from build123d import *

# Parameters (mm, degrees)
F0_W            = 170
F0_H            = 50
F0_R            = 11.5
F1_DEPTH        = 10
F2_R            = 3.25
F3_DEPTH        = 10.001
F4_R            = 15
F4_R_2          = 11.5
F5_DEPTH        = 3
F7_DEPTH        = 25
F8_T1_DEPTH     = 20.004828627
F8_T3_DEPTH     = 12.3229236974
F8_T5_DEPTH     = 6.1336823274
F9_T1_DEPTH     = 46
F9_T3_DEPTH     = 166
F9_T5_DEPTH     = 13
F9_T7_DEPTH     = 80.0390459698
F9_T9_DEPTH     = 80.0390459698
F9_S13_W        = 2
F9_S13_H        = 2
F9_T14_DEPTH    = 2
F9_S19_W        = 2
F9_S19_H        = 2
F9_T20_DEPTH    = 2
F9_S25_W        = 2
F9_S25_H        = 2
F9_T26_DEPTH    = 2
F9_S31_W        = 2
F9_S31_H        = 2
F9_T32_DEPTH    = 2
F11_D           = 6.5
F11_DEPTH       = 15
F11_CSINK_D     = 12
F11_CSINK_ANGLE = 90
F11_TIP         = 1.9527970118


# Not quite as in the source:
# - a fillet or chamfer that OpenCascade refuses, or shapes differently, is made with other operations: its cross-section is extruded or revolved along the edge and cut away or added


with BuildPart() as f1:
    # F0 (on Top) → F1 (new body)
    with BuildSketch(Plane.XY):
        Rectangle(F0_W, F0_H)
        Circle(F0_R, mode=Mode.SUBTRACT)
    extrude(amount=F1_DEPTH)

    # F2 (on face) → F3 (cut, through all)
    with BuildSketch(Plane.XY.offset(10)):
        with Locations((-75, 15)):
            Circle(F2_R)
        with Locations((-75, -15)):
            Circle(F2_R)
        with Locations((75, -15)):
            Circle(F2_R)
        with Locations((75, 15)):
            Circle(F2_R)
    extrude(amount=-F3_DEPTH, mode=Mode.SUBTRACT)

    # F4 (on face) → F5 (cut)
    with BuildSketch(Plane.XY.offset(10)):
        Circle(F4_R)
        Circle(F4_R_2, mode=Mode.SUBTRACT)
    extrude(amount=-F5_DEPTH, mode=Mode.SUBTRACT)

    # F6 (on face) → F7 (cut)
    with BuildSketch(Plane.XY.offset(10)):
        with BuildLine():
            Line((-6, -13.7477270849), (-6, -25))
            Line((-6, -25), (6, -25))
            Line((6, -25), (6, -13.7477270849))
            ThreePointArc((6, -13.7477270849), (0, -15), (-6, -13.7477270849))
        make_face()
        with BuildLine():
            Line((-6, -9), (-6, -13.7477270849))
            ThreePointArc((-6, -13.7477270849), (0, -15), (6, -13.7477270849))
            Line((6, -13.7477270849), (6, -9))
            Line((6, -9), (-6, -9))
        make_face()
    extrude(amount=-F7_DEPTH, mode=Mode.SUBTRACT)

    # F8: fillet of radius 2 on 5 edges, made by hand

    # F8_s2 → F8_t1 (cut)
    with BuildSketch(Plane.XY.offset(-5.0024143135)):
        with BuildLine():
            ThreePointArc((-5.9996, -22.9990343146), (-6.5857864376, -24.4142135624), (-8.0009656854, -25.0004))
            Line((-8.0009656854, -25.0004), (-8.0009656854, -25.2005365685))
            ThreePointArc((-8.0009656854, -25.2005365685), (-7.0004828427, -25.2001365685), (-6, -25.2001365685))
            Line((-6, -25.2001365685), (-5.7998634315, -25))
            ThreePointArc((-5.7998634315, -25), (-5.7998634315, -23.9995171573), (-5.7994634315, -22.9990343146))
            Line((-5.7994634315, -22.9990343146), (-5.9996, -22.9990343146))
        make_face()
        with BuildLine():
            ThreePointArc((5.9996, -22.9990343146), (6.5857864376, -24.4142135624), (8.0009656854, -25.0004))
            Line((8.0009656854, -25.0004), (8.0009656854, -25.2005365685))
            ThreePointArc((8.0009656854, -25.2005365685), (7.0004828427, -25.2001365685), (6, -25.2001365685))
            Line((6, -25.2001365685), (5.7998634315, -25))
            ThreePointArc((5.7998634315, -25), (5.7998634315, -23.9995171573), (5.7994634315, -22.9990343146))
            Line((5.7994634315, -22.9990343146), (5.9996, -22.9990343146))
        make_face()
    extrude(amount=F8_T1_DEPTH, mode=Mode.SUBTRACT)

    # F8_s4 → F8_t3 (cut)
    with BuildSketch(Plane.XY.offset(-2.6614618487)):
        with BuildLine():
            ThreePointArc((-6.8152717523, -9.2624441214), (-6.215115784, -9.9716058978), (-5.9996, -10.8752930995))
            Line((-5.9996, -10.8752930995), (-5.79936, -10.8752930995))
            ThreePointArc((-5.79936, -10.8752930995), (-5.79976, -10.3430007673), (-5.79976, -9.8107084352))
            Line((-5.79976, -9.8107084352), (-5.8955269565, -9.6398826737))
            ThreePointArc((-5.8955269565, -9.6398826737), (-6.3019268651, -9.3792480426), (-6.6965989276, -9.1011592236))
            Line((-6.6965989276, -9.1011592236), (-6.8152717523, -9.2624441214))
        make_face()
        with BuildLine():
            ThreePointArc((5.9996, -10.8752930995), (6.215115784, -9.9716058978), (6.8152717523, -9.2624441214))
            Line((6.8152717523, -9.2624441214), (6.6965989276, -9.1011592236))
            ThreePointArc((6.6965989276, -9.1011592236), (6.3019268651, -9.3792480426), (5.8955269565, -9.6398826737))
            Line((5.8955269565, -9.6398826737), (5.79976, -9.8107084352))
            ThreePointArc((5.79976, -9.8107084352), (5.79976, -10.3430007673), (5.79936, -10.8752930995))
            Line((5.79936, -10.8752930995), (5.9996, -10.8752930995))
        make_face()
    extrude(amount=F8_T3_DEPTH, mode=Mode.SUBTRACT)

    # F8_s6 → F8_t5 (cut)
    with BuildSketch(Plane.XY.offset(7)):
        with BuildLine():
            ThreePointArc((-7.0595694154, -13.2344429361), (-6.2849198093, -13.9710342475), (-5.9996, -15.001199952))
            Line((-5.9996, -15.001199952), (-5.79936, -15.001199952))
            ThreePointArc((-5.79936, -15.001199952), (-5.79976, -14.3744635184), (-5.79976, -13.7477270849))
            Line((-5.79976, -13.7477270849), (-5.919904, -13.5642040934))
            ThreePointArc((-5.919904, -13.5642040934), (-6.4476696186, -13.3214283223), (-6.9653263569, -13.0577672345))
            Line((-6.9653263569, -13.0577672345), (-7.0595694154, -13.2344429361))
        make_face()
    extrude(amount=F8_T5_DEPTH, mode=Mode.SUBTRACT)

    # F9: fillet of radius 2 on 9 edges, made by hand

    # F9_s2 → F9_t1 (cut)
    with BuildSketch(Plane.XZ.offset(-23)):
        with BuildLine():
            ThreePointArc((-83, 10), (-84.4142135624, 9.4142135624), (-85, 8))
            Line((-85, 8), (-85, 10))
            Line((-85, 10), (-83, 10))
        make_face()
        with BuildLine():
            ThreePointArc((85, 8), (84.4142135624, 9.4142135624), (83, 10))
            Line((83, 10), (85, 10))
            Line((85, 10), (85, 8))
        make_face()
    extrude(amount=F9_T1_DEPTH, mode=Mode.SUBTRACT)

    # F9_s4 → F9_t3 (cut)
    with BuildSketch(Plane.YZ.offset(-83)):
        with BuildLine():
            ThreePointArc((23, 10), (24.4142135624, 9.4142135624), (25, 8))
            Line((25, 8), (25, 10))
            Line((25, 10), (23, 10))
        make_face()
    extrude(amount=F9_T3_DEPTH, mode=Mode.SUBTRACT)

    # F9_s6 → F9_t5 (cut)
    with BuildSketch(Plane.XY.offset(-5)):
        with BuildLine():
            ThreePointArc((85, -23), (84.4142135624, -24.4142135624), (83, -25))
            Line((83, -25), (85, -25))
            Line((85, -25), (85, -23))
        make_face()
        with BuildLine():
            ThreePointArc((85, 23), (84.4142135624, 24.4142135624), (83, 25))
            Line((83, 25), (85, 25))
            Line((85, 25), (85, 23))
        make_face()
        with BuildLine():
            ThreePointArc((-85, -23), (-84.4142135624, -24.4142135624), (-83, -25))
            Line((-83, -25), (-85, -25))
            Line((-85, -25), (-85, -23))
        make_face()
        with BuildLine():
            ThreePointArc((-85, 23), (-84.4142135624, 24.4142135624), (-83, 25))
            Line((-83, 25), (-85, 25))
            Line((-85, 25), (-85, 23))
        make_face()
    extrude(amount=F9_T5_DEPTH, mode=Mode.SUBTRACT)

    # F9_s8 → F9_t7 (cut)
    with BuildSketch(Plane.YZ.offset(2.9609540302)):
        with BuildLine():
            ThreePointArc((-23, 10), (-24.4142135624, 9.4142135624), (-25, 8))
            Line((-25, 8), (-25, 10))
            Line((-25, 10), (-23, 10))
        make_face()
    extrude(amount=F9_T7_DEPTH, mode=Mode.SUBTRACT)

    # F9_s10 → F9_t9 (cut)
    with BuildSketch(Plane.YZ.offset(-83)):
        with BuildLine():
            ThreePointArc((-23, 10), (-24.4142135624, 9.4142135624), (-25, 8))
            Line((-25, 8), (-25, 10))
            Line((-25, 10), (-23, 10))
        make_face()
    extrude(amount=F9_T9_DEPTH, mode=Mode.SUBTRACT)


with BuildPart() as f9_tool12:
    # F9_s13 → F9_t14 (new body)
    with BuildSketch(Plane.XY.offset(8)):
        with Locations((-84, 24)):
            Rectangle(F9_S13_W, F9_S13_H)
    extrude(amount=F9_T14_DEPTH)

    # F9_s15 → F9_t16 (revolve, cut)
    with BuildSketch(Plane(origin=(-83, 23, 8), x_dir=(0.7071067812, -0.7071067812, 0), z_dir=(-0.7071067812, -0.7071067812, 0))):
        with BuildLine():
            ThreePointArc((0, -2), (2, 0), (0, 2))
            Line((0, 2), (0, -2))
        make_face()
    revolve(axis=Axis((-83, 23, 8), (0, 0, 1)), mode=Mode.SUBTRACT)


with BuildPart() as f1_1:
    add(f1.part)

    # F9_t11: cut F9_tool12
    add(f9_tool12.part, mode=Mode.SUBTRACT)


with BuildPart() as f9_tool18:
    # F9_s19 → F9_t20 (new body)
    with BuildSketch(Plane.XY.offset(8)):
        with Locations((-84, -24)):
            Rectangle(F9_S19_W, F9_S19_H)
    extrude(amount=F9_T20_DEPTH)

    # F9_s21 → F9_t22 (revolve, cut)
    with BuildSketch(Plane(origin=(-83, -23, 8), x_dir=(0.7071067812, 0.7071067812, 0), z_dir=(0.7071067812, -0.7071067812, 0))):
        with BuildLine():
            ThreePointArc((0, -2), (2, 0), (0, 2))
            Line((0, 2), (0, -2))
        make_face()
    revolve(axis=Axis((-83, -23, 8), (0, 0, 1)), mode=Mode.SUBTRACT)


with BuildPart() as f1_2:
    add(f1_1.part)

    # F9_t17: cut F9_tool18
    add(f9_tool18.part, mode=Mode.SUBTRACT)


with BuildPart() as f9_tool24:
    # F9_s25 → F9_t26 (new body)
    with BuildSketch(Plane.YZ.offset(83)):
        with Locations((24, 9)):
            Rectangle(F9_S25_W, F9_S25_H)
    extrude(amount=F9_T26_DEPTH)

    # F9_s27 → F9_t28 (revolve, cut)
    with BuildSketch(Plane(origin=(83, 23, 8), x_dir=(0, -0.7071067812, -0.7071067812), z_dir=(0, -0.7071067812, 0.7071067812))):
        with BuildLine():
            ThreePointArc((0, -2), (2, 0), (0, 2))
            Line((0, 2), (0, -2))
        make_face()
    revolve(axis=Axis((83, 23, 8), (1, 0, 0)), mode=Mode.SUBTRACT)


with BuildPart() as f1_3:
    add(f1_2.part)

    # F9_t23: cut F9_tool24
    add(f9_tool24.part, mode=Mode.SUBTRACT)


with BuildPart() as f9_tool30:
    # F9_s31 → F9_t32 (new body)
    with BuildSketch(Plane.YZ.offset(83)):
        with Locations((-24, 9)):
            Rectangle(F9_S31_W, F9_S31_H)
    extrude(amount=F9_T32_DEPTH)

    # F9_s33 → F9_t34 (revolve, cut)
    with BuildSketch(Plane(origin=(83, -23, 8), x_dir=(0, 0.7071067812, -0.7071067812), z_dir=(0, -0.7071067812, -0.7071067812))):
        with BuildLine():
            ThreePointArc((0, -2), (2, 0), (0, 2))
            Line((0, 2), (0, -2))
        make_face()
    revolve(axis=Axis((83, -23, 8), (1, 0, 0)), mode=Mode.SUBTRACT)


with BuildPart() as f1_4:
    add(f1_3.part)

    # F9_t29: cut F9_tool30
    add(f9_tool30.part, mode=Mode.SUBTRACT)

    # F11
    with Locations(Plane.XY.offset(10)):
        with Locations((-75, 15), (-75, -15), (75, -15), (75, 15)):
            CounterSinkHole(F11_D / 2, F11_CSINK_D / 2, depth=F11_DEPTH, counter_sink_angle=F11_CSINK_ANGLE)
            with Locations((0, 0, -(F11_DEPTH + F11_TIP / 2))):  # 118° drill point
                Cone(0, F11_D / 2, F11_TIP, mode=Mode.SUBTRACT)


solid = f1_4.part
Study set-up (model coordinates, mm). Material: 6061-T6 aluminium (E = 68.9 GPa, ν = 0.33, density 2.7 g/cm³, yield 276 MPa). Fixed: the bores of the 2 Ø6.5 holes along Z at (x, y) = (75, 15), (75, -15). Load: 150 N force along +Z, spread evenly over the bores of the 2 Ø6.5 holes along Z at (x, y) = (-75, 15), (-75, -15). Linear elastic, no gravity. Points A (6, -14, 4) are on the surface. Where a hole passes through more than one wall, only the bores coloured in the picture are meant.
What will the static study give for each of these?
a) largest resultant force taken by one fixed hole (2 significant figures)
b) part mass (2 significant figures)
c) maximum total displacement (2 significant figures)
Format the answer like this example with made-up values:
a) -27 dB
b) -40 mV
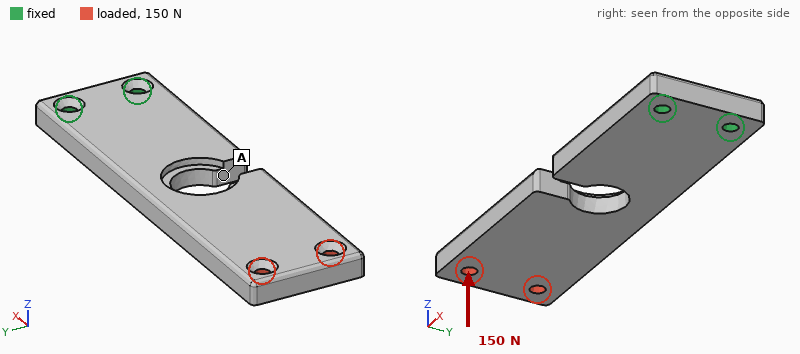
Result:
a) 88 N
b) 210 g
c) 1.2 mm
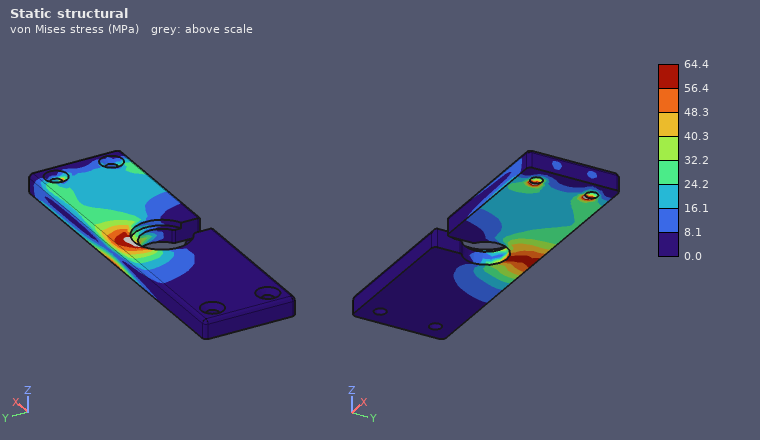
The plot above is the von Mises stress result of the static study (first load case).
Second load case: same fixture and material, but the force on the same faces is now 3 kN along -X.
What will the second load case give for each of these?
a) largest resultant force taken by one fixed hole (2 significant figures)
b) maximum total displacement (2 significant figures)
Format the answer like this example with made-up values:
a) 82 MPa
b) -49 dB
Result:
a) 1.5 kN
b) 1.1 mm
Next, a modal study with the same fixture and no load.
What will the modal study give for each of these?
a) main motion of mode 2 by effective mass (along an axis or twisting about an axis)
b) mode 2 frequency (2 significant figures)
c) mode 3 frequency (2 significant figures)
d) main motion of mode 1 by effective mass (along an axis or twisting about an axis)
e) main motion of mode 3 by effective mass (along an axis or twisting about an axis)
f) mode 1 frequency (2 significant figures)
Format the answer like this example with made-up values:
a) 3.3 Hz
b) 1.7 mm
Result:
a) along Y
b) 570 Hz
c) 1200 Hz
d) along Z
e) twisting about X
f) 260 Hz
